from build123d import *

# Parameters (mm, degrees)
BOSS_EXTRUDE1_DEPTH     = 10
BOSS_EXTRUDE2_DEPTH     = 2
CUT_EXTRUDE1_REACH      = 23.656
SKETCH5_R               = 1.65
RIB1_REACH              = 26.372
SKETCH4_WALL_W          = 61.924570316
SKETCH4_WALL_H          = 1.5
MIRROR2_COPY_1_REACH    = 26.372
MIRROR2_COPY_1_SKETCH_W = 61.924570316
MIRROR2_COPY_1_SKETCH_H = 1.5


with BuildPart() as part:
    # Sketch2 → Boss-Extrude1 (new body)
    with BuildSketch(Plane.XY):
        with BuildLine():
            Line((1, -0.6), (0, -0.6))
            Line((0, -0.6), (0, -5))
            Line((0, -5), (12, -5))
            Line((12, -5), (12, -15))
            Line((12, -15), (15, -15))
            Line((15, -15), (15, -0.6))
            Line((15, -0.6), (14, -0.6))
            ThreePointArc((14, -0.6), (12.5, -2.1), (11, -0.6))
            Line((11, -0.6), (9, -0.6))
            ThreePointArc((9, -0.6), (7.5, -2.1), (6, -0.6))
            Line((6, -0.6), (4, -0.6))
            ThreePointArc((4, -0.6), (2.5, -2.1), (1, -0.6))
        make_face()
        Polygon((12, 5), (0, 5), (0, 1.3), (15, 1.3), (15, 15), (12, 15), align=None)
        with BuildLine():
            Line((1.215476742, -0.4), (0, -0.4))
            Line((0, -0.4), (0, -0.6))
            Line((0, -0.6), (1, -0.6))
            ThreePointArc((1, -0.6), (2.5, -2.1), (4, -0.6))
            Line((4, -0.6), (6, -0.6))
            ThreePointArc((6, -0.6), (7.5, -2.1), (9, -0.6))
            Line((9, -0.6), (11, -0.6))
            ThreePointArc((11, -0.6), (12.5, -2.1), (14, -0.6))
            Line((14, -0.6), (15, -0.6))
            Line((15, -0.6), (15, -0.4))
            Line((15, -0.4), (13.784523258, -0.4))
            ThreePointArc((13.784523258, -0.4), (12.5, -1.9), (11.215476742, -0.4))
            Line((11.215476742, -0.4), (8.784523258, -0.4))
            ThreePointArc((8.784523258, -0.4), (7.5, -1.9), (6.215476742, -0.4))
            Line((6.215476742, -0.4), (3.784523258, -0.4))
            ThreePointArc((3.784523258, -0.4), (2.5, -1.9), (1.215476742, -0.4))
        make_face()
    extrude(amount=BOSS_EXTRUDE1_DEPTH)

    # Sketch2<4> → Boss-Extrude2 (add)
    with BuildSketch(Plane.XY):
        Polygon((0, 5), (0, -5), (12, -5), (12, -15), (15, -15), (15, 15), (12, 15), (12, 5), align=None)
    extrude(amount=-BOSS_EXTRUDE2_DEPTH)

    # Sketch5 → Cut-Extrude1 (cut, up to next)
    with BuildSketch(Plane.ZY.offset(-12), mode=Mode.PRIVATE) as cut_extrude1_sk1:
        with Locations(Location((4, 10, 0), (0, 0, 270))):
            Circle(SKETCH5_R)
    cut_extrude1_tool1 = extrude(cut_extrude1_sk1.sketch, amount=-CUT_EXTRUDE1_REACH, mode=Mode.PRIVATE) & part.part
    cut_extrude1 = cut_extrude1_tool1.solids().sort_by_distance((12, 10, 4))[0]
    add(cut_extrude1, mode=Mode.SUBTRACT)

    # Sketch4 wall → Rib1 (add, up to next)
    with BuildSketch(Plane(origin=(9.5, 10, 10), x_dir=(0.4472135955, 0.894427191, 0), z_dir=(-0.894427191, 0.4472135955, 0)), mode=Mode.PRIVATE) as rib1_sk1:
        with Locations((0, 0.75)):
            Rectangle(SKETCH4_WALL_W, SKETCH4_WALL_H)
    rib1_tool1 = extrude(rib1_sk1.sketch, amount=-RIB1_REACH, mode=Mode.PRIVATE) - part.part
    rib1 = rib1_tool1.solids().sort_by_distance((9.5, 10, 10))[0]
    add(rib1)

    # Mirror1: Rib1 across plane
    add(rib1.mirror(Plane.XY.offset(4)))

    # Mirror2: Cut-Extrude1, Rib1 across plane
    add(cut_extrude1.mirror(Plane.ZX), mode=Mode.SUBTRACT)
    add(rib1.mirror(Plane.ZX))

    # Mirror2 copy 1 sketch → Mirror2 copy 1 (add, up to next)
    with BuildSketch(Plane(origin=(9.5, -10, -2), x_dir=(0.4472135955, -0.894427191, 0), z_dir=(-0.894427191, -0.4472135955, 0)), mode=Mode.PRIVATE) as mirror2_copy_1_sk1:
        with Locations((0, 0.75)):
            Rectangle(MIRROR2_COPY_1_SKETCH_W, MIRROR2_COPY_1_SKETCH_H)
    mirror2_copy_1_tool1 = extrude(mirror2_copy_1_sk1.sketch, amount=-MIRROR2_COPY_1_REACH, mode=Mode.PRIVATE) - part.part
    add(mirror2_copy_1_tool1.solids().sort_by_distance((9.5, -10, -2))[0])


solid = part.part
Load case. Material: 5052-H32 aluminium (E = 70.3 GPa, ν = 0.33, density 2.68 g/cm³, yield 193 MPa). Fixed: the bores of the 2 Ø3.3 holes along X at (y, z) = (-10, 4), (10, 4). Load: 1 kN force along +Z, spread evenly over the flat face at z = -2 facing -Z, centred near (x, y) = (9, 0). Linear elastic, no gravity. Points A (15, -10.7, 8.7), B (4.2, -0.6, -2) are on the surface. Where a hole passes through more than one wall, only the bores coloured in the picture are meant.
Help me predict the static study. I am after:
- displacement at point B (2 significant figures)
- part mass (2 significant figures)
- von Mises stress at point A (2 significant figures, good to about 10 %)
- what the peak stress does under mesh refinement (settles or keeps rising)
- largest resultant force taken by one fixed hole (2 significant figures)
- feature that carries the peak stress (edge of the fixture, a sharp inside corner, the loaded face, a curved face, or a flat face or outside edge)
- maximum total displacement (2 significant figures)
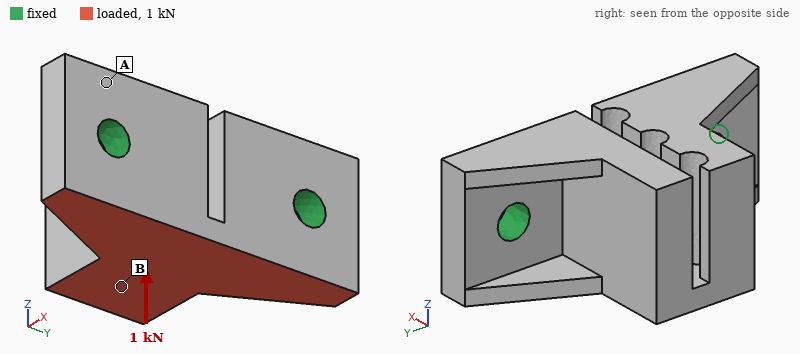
31 µm
6.1 g
31 MPa
keeps rising
530 N
edge of the fixture
41 µm
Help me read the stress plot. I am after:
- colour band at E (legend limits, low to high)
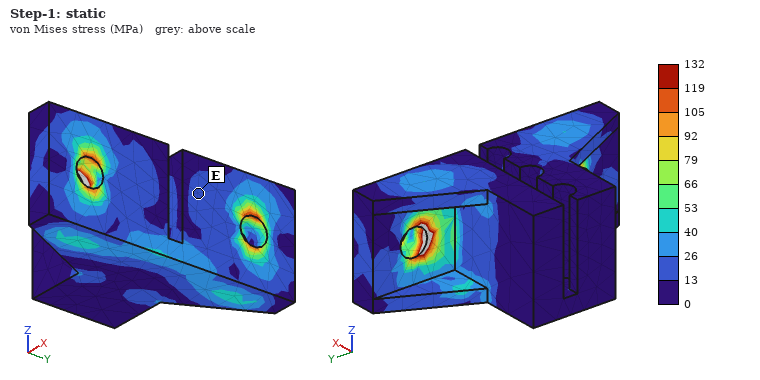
13 to 26 MPa
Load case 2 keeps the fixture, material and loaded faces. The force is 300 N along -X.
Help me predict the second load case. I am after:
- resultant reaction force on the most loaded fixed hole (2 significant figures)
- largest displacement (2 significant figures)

150 N
13 µm
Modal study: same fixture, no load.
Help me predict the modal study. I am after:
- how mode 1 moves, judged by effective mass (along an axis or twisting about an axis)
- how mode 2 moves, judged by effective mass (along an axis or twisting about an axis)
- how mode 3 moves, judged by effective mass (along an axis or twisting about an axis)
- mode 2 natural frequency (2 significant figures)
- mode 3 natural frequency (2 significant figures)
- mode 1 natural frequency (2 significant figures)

along Z
along Y
along X
18 kHz
21 kHz
12 kHz
